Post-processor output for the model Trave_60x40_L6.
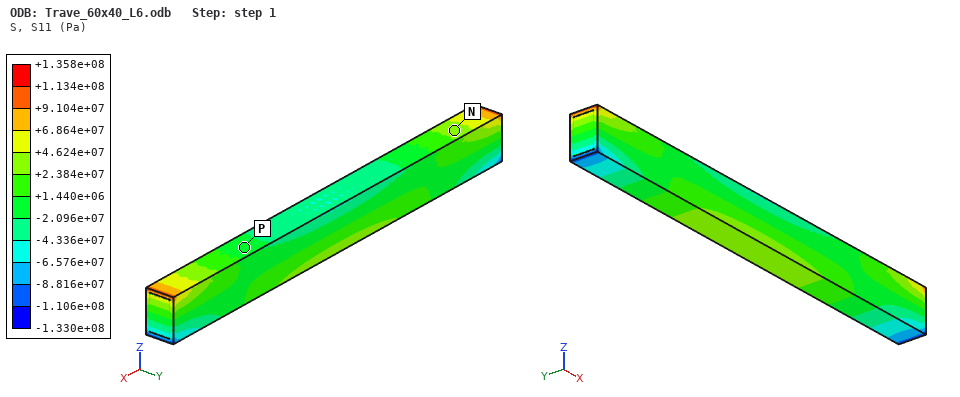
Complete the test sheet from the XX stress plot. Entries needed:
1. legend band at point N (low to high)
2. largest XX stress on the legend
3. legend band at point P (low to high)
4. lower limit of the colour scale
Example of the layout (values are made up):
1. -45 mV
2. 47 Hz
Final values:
1. +2.384e+07 to +4.624e+07 Pa
2. +1.358e+08 Pa
3. -2.096e+07 to +1.440e+06 Pa
4. -1.330e+08 Pa
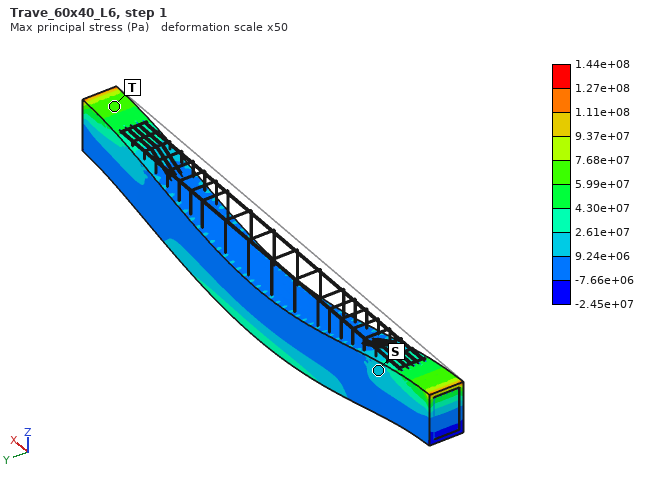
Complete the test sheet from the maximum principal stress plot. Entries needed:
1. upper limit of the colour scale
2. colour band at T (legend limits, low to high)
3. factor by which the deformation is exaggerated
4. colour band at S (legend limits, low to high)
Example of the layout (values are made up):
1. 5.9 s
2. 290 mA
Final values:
1. 1.44e+08 Pa
2. 5.99e+07 to 7.68e+07 Pa
3. 50
4. 9.24e+06 to 2.61e+07 Pa
